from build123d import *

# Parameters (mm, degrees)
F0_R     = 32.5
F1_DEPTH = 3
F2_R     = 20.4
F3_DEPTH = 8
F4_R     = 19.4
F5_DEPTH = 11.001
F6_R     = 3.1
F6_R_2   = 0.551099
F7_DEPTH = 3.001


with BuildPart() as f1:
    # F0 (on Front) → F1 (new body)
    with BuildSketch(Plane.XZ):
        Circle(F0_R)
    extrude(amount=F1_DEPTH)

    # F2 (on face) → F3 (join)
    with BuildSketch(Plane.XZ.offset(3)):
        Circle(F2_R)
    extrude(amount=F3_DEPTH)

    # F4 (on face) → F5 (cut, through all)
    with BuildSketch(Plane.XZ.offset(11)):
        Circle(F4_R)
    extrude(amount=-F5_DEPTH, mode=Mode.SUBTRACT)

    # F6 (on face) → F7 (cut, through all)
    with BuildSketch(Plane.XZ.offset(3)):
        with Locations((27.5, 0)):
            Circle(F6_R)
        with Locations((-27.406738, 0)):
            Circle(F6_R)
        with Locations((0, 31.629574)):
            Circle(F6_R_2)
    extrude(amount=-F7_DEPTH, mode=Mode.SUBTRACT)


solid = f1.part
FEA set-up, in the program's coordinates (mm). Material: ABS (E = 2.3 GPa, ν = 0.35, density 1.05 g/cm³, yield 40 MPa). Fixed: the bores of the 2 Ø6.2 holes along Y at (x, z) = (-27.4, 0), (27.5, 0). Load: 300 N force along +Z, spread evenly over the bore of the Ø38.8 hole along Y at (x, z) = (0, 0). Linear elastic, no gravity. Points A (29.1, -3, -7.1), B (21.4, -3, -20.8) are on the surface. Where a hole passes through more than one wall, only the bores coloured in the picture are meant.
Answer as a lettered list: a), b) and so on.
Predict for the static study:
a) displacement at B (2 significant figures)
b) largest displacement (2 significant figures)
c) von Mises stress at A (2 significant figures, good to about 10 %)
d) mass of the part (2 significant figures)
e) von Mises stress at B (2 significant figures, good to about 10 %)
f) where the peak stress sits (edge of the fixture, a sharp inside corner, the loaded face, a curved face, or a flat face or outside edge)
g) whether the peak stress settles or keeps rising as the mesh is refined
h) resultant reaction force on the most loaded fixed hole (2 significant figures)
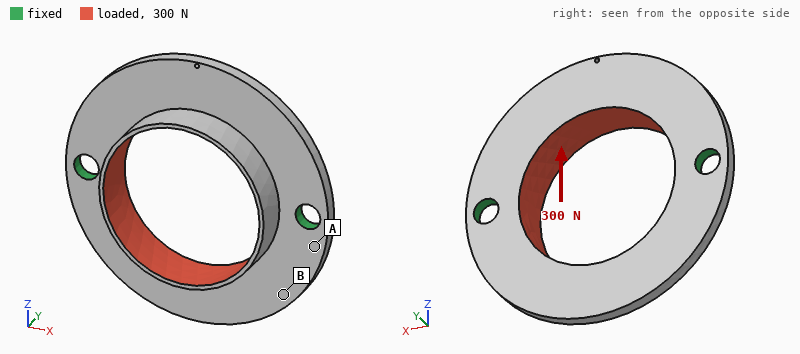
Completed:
a) 0.41 mm
b) 0.93 mm
c) 9.3 MPa
d) 7.6 g
e) 2.7 MPa
f) edge of the fixture
g) keeps rising
h) 150 N
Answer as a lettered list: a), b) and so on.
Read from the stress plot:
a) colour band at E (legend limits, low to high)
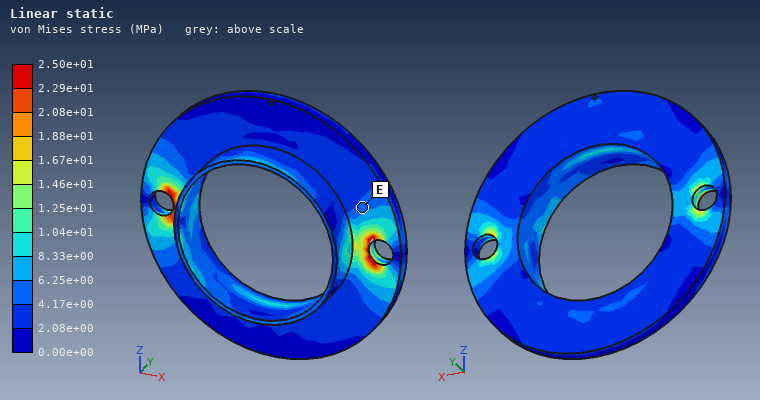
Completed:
a) 4.17e+00 to 6.25e+00 MPa
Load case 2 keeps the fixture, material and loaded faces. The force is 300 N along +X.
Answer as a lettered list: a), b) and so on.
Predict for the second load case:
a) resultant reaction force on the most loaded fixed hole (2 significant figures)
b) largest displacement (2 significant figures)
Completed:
a) 150 N
b) 0.14 mm
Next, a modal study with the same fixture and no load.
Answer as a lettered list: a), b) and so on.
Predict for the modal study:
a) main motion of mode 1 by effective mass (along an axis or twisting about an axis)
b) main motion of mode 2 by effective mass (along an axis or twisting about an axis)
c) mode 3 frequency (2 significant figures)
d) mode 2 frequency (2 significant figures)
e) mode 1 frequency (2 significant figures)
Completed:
a) twisting about X
b) along Y
c) 1800 Hz
d) 800 Hz
e) 670 Hz
